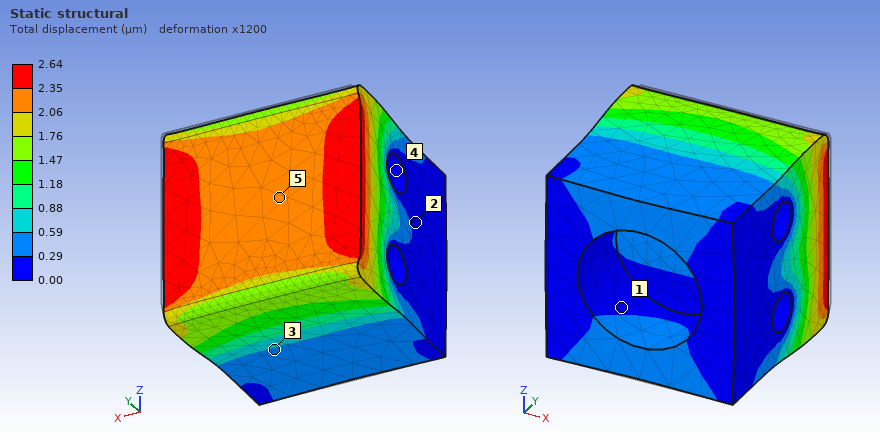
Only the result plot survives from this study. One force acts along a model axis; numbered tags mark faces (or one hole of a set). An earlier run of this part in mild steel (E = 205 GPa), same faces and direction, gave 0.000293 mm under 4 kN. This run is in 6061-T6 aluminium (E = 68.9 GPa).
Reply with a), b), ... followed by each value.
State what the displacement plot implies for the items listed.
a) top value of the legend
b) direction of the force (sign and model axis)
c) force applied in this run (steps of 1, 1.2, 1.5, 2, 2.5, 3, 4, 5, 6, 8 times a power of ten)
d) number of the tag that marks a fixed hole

a) 2.64 µm
b) -Y
c) 12 kN
d) 4
